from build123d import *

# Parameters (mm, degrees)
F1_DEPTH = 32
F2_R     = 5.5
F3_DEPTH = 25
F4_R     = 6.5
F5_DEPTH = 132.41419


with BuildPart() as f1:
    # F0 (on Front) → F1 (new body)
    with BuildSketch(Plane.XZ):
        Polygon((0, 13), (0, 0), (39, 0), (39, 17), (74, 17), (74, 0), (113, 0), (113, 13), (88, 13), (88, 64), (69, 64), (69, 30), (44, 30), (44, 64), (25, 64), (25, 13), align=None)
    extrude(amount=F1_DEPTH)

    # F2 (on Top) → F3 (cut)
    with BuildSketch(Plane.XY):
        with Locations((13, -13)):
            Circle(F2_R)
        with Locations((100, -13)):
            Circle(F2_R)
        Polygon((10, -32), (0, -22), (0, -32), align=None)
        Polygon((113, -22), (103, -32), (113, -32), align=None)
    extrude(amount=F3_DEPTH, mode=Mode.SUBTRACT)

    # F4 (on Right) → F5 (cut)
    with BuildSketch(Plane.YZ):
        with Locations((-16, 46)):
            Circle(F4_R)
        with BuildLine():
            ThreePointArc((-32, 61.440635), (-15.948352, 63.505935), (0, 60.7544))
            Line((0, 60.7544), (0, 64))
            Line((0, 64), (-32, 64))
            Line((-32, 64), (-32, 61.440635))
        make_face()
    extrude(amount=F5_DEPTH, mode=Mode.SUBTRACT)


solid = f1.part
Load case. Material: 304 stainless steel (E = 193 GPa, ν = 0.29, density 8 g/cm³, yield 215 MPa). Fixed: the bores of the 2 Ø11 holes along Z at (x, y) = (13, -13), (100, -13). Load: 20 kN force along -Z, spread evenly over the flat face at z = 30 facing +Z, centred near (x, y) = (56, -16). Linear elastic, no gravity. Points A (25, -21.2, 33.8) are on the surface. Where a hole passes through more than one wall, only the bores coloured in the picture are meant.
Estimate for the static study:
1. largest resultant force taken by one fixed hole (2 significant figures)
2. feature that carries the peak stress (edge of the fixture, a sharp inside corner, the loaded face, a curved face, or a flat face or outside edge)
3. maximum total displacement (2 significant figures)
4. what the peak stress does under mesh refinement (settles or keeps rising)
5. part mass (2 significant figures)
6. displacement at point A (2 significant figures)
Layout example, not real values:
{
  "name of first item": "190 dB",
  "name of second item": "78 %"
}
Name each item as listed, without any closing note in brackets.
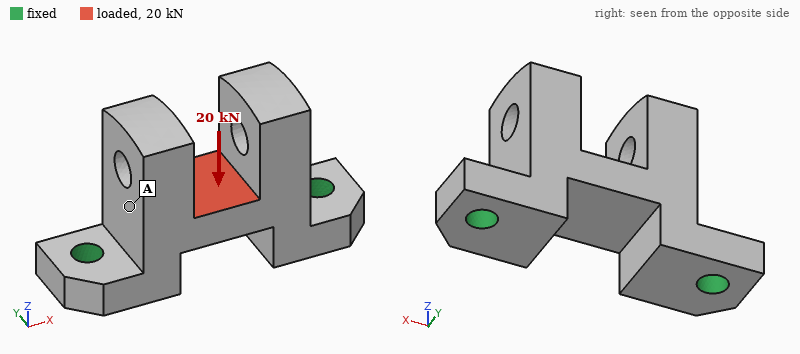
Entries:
{
  "largest resultant force taken by one fixed hole": "15 kN",
  "feature that carries the peak stress": "edge of the fixture",
  "maximum total displacement": "37 µm",
  "what the peak stress does under mesh refinement": "keeps rising",
  "part mass": "750 g",
  "displacement at point A": "13 µm"
}
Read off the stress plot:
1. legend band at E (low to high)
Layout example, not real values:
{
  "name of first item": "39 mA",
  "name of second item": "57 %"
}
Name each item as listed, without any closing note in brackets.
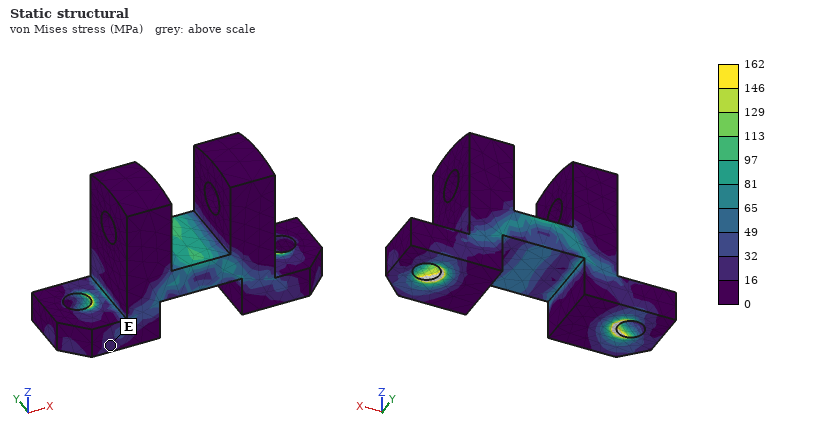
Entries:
{
  "legend band at E": "16 to 32 MPa"
}
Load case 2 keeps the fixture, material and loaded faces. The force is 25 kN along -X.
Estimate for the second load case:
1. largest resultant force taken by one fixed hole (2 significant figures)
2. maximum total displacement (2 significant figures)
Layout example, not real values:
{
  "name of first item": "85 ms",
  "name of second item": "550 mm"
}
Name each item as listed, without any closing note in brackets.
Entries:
{
  "largest resultant force taken by one fixed hole": "15 kN",
  "maximum total displacement": "23 µm"
}
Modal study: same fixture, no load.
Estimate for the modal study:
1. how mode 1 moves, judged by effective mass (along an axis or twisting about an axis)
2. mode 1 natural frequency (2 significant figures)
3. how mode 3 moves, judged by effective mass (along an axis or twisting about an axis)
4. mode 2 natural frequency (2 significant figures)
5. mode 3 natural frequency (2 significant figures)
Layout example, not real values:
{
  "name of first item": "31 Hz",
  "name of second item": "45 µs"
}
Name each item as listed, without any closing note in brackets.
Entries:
{
  "how mode 1 moves, judged by effective mass": "along Y",
  "mode 1 natural frequency": "2700 Hz",
  "how mode 3 moves, judged by effective mass": "along X",
  "mode 2 natural frequency": "4500 Hz",
  "mode 3 natural frequency": "5500 Hz"
}
